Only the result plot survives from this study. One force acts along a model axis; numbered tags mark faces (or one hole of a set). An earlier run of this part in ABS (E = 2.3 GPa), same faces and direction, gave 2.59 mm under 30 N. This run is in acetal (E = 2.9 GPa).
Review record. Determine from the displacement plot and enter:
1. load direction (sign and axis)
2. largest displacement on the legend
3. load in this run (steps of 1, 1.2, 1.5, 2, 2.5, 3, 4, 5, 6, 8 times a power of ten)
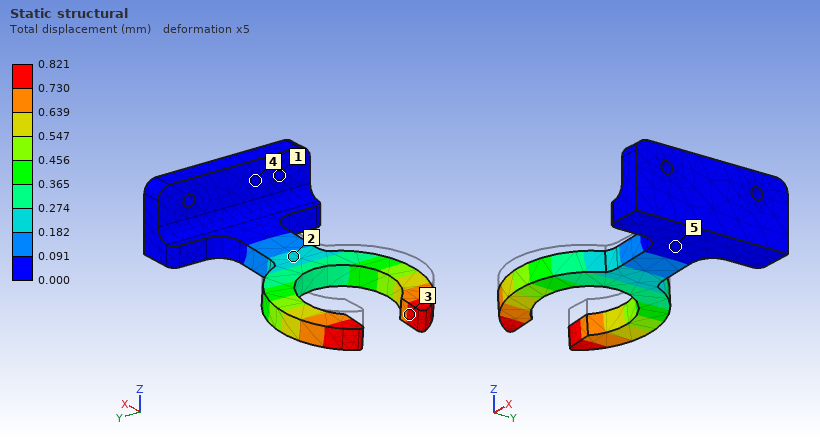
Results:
-Z
0.821 mm
12 N
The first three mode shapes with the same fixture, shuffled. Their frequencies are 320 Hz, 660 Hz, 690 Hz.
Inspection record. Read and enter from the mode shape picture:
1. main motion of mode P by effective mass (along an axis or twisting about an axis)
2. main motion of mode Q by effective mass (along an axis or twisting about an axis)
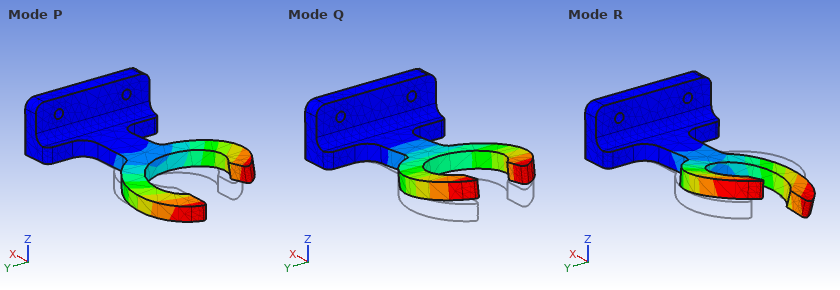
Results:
along Y
along Z
